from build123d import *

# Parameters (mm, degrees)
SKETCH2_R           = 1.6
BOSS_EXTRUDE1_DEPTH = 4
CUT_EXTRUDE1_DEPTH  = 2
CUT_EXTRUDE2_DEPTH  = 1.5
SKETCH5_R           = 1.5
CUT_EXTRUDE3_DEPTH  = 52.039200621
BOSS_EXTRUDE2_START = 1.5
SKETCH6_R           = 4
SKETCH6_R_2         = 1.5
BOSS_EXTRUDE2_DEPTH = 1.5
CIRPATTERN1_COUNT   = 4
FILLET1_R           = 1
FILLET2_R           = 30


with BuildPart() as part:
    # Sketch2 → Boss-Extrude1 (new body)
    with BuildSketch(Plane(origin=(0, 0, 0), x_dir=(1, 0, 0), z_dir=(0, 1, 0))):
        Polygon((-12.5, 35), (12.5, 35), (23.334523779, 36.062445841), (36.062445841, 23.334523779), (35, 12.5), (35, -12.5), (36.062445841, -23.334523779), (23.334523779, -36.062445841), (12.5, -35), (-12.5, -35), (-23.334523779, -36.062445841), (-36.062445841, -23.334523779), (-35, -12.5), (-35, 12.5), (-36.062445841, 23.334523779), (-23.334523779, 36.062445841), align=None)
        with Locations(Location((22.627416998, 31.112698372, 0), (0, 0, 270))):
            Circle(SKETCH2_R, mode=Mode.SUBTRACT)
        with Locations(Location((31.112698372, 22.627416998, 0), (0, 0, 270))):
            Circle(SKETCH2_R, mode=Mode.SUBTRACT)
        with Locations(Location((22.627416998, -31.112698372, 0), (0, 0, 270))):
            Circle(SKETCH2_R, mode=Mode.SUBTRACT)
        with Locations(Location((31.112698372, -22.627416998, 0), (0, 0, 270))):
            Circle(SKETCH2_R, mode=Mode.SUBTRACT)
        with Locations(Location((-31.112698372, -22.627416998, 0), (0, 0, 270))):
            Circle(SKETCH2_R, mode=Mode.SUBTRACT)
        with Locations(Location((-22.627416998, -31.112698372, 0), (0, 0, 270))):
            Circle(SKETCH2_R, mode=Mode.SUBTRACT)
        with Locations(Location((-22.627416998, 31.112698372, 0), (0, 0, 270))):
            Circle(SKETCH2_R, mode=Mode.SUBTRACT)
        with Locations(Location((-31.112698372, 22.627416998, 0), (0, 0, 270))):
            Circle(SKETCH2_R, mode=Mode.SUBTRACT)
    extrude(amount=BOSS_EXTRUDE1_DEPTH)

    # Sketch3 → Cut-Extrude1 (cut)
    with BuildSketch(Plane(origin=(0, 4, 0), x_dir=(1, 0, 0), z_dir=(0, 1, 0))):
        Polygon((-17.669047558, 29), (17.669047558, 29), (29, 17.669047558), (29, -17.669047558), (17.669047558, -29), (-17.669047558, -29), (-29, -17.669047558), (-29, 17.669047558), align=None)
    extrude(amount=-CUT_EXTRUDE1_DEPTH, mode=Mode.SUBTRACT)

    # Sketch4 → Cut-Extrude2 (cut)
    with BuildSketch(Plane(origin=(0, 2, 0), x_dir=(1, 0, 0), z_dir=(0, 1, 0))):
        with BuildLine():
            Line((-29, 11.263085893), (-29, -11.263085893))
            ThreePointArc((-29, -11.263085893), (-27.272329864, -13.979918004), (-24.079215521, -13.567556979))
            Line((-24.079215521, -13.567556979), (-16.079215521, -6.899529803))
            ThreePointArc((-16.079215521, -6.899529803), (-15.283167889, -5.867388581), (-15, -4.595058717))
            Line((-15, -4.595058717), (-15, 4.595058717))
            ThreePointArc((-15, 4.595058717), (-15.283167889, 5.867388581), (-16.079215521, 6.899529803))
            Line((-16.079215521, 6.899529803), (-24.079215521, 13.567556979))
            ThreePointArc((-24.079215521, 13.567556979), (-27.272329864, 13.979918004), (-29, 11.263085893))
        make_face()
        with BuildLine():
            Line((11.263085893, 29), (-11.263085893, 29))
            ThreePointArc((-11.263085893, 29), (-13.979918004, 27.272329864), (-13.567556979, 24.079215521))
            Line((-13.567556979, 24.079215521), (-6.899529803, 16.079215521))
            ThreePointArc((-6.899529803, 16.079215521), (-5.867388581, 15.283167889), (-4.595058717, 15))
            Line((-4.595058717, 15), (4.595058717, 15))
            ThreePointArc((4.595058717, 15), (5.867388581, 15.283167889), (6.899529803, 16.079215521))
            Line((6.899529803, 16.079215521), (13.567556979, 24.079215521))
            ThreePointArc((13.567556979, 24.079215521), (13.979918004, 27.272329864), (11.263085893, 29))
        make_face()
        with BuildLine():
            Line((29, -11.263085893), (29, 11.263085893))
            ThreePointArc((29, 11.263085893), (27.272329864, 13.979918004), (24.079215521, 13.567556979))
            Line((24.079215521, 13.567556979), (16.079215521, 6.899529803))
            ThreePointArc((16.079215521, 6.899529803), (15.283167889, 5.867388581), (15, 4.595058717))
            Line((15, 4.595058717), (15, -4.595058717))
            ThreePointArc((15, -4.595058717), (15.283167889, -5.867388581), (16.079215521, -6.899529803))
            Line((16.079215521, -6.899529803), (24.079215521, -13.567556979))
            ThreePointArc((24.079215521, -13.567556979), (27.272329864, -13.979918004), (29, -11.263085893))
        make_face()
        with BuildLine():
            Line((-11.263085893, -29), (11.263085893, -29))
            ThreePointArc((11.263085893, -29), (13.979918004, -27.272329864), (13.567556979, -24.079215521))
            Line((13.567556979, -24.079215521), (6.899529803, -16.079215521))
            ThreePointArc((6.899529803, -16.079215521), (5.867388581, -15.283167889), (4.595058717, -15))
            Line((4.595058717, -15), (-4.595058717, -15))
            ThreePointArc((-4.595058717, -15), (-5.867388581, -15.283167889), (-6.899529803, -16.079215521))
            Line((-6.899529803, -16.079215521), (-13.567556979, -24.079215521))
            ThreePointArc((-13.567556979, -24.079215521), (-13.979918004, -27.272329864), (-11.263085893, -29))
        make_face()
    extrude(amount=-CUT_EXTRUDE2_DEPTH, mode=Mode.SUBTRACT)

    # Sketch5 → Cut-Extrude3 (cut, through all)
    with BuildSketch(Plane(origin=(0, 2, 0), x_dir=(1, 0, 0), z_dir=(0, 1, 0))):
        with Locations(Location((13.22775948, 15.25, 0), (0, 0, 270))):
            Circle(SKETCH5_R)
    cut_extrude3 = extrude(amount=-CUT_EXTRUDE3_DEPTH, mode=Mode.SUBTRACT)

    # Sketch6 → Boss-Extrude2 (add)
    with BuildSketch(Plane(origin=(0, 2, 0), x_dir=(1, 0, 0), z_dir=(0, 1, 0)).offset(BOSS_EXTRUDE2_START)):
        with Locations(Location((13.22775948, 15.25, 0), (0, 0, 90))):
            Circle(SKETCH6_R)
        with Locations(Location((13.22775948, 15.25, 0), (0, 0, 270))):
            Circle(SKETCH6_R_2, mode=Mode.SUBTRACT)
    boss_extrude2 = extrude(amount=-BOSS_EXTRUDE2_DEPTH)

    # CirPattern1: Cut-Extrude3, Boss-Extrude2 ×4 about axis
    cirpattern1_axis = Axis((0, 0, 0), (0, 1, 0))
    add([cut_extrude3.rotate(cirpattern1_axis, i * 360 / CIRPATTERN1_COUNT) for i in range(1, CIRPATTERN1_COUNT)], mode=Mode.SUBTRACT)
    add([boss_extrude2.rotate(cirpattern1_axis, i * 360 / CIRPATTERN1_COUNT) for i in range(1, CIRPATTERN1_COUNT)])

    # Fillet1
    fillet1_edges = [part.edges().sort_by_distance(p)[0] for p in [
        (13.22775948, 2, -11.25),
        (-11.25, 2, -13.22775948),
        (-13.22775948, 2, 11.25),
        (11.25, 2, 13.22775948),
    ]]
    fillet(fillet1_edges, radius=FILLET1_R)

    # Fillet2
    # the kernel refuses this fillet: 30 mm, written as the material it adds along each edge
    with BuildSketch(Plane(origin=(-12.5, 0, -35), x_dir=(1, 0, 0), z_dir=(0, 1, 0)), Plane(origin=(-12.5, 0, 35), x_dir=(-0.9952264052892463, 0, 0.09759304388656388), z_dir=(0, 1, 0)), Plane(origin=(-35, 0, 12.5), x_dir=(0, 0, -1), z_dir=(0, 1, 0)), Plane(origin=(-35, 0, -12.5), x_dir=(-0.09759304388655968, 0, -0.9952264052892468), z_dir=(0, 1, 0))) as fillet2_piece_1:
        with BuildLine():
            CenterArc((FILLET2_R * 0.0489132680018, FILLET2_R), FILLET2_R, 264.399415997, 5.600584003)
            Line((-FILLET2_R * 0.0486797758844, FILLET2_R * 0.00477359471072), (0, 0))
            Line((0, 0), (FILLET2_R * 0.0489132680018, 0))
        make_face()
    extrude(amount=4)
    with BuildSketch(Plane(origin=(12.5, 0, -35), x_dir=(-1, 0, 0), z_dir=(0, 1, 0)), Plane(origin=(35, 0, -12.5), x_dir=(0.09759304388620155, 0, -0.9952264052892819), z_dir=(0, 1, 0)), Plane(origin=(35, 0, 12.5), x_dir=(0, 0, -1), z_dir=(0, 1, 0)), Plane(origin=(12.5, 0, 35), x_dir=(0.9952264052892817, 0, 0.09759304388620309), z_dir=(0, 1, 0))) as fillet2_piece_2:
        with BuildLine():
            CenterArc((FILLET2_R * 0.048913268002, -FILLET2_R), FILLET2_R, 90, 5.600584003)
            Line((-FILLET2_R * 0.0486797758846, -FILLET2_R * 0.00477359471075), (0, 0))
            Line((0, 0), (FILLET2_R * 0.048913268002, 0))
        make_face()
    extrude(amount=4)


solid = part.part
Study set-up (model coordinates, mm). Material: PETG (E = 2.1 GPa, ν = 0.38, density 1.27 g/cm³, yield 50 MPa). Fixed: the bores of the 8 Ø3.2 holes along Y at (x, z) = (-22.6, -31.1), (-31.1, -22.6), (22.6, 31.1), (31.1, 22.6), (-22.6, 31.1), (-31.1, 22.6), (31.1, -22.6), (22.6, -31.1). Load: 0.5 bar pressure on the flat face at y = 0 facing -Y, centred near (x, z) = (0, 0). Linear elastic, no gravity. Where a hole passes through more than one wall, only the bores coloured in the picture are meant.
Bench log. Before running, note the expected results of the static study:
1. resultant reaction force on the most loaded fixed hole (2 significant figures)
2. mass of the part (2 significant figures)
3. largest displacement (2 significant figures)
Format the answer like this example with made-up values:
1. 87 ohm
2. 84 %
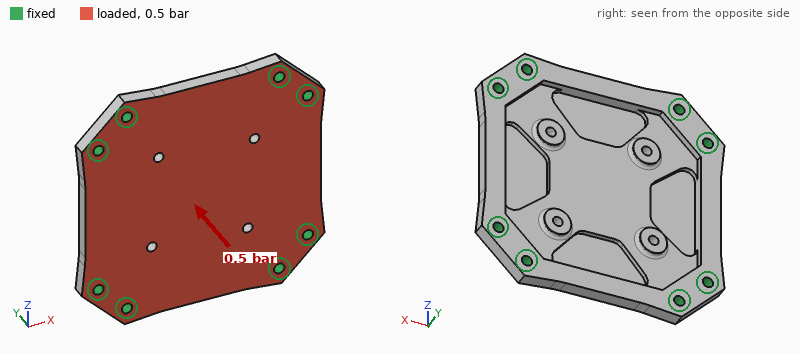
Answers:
1. 35 N
2. 14 g
3. 1.2 mm
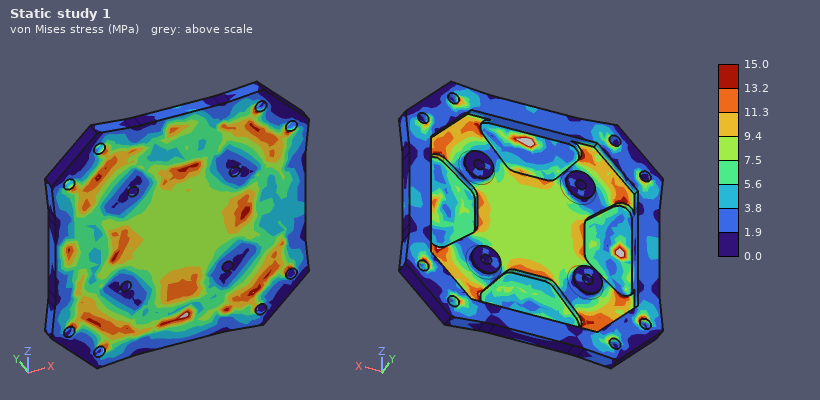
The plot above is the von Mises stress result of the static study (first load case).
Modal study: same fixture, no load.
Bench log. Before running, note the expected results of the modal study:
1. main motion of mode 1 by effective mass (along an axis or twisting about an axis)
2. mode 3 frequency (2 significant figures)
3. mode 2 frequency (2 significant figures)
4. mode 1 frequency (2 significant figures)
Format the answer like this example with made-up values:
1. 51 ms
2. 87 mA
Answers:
1. along Y
2. 1800 Hz
3. 1800 Hz
4. 850 Hz
